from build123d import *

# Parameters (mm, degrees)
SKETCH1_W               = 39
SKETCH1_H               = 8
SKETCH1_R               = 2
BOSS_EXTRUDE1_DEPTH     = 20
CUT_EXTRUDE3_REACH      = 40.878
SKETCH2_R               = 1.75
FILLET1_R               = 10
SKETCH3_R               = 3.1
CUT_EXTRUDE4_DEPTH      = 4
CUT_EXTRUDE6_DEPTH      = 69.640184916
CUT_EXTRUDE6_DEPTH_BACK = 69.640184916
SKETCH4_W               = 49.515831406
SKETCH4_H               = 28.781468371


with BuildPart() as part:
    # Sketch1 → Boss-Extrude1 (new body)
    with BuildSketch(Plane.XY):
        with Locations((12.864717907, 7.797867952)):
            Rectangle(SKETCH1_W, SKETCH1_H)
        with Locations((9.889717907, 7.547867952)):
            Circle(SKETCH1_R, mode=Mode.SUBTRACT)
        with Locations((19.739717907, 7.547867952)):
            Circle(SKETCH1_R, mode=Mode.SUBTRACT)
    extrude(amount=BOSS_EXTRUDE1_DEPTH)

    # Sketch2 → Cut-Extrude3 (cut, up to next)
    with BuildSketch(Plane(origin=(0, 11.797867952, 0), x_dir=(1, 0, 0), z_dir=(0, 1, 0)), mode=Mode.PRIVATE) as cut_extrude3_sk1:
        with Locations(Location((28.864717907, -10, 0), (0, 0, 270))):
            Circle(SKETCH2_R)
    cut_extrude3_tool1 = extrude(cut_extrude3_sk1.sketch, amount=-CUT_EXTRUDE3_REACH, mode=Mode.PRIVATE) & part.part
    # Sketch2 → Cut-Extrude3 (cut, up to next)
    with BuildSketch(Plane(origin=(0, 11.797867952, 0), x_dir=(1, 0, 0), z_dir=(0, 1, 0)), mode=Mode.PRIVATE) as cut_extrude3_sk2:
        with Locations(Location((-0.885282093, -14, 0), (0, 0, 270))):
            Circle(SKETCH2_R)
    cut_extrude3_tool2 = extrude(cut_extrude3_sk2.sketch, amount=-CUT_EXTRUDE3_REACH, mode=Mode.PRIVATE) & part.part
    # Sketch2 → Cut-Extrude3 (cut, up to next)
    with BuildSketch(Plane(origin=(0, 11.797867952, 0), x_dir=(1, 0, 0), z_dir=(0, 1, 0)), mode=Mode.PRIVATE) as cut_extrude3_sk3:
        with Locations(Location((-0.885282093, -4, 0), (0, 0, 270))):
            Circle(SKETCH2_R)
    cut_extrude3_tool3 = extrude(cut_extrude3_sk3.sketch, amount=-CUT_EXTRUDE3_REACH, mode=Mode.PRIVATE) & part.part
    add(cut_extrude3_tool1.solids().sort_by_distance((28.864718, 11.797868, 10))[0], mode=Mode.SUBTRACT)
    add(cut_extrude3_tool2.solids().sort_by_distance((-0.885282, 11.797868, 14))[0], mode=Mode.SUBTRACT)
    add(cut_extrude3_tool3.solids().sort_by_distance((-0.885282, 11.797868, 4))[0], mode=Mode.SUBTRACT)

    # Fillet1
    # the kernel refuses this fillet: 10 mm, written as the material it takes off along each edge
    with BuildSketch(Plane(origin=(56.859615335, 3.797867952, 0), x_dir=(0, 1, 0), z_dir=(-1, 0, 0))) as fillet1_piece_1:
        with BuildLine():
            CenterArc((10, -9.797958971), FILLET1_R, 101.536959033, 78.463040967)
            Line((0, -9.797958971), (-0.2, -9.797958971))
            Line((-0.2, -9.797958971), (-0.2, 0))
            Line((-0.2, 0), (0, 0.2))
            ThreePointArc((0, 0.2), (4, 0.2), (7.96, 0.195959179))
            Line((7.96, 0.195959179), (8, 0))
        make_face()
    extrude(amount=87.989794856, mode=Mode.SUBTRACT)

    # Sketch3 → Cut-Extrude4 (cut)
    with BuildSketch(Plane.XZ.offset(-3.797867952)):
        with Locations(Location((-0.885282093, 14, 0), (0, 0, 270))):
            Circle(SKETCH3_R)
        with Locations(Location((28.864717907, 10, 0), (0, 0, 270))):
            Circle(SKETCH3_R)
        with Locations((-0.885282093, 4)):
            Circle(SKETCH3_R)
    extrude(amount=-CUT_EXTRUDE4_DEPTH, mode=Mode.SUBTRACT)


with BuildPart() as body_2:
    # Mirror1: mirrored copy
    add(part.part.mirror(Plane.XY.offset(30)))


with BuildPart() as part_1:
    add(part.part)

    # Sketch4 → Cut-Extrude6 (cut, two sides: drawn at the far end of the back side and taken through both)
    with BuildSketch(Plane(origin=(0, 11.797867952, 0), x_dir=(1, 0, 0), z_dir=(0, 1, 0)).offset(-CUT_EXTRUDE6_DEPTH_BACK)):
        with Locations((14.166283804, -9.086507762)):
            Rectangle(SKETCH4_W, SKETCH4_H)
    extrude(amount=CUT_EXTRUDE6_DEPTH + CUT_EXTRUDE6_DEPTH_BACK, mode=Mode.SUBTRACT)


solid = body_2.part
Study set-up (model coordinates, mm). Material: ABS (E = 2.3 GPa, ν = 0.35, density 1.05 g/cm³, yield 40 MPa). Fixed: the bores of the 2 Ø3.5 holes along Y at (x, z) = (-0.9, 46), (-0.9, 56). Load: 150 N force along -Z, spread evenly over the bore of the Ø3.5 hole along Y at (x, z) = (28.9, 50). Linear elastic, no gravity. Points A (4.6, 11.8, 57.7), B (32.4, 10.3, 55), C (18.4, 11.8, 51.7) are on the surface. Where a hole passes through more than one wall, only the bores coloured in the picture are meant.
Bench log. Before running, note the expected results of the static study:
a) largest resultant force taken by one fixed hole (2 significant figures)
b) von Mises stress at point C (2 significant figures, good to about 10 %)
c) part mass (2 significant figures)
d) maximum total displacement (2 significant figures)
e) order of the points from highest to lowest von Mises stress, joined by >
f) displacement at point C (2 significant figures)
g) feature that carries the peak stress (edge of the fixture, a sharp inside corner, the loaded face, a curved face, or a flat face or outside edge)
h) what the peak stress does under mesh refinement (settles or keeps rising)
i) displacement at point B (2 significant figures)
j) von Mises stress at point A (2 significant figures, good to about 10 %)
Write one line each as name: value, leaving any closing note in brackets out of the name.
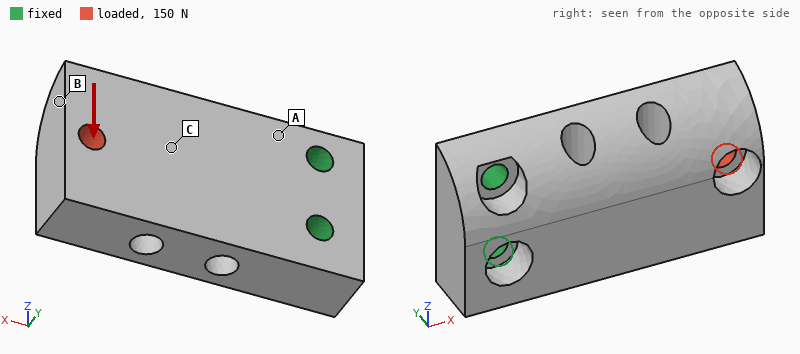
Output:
largest resultant force taken by one fixed hole: 370 N
von Mises stress at point C: 6.0 MPa
part mass: 4.8 g
maximum total displacement: 0.44 mm
order of the points from highest to lowest von Mises stress, joined by >: A > C > B
displacement at point C: 0.19 mm
feature that carries the peak stress: edge of the fixture
what the peak stress does under mesh refinement: keeps rising
displacement at point B: 0.41 mm
von Mises stress at point A: 12 MPa
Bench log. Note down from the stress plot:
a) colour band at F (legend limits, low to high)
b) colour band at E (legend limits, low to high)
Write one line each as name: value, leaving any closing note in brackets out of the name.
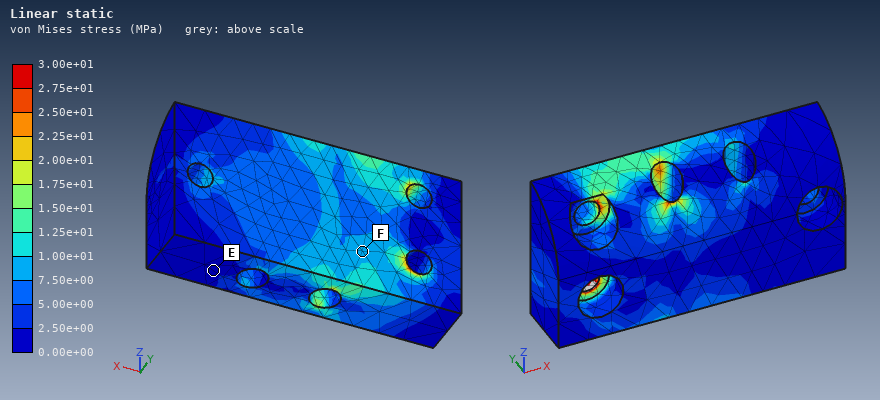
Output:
colour band at F: 7.50e+00 to 1.00e+01 MPa
colour band at E: 0.00e+00 to 2.50e+00 MPa
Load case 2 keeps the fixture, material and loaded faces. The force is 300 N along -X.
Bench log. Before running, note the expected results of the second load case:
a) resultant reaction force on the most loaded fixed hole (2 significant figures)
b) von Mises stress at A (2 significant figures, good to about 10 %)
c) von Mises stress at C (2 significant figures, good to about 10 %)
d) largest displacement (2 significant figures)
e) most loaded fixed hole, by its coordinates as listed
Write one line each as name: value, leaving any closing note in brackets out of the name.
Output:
resultant reaction force on the most loaded fixed hole: 170 N
von Mises stress at A: 5.8 MPa
von Mises stress at C: 6.2 MPa
largest displacement: 0.17 mm
most loaded fixed hole, by its coordinates as listed: (-0.9, 46)
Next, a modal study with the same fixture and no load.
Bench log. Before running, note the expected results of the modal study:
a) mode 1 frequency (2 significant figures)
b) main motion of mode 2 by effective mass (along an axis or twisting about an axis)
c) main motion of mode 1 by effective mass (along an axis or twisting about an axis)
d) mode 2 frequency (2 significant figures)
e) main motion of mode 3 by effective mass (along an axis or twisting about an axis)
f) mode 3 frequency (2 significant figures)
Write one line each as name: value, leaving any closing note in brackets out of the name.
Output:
mode 1 frequency: 1200 Hz
main motion of mode 2 by effective mass: along Z
main motion of mode 1 by effective mass: along Y
mode 2 frequency: 2800 Hz
main motion of mode 3 by effective mass: twisting about X
mode 3 frequency: 4300 Hz
